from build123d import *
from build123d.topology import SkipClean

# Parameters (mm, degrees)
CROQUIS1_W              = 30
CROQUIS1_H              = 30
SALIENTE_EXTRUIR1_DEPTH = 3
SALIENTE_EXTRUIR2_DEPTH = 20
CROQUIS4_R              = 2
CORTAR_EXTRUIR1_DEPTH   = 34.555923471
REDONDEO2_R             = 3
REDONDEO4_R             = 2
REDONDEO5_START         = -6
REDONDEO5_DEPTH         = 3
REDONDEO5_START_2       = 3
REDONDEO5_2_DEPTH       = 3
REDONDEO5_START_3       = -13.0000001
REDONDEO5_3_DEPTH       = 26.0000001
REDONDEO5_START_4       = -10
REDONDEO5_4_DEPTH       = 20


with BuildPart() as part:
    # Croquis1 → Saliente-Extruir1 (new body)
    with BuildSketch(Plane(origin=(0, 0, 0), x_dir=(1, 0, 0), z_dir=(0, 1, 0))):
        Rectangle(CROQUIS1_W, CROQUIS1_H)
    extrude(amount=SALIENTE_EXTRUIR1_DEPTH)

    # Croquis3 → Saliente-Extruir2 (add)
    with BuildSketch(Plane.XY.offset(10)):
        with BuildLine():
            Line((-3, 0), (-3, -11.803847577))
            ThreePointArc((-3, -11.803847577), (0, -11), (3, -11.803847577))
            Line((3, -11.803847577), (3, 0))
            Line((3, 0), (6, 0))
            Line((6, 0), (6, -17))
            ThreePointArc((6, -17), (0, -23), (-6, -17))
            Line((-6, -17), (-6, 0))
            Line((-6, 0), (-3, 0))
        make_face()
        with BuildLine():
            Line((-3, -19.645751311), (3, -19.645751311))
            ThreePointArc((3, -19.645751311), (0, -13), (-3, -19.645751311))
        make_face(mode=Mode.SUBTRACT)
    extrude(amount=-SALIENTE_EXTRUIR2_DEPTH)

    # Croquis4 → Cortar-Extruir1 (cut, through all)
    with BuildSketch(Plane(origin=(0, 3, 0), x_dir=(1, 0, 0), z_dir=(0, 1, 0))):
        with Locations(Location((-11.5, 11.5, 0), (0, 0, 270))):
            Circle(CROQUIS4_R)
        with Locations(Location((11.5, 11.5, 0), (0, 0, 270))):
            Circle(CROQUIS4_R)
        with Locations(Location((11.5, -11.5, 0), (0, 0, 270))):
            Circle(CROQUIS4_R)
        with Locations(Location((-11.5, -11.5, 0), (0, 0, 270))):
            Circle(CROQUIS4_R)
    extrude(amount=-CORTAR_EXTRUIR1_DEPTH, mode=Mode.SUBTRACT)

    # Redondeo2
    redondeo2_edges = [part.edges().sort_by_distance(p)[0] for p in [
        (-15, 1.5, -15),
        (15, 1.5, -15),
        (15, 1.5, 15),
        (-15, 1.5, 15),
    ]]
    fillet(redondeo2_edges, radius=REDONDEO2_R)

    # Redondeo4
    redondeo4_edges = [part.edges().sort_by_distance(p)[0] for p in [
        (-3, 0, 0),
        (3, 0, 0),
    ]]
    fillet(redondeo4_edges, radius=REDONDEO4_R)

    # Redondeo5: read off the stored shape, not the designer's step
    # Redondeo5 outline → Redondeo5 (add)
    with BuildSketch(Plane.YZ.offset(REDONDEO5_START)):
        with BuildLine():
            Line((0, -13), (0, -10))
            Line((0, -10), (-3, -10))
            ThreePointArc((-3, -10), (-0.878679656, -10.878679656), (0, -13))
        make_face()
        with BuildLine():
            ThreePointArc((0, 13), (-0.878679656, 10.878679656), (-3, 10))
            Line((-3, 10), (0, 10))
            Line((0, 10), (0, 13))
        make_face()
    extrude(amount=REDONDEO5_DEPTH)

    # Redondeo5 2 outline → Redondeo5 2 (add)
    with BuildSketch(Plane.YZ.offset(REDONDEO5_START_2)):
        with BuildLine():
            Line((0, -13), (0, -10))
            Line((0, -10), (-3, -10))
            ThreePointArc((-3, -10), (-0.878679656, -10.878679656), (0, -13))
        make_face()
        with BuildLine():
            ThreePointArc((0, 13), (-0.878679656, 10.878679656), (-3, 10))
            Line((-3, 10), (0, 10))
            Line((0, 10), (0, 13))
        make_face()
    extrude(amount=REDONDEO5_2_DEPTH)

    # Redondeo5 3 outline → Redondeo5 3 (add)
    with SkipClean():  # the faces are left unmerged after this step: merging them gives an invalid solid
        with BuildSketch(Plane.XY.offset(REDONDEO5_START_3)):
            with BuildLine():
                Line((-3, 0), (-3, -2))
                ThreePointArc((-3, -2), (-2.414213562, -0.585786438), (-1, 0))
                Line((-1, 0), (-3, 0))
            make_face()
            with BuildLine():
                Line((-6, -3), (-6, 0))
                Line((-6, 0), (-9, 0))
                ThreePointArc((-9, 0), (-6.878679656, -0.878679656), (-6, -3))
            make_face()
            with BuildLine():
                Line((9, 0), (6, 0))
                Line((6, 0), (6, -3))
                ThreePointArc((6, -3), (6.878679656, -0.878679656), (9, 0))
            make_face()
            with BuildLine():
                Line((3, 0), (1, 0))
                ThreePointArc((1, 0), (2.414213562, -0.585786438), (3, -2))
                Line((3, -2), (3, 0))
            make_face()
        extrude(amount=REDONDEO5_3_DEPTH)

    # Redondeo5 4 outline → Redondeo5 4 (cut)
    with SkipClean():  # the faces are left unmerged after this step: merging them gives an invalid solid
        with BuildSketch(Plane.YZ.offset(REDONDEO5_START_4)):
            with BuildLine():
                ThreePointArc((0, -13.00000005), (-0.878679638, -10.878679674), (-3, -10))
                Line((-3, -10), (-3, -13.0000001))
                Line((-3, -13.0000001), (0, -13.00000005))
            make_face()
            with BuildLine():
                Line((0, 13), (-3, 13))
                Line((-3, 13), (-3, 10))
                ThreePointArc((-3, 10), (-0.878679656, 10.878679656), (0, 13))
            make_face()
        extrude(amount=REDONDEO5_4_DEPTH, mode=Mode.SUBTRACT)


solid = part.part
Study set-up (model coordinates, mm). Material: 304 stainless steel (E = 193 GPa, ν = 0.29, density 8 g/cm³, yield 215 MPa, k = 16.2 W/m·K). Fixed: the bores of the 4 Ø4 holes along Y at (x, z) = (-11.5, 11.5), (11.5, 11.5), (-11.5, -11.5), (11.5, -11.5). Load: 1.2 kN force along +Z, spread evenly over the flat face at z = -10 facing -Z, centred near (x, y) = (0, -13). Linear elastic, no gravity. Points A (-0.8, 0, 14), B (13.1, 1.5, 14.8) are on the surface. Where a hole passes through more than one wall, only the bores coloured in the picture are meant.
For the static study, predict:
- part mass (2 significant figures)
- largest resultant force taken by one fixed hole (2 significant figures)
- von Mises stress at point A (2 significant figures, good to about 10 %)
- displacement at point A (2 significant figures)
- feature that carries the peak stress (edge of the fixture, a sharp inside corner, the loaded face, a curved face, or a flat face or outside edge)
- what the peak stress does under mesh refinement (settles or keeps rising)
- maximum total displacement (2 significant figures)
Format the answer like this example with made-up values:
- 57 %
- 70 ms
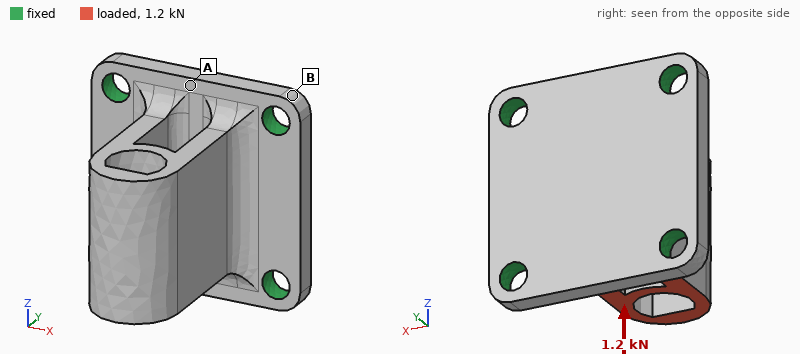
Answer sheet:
- 45 g
- 530 N
- 27 MPa
- 4.1 µm
- edge of the fixture
- keeps rising
- 13 µm
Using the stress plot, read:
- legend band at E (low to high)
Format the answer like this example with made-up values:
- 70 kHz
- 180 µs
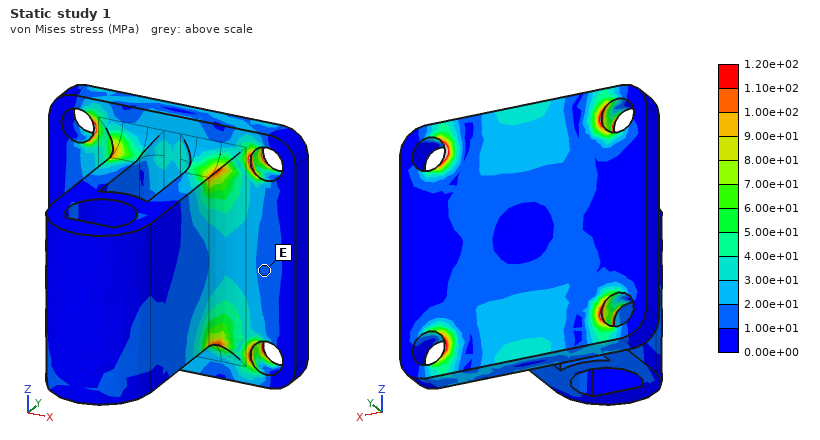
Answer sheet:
- 1.00e+01 to 2.00e+01 MPa
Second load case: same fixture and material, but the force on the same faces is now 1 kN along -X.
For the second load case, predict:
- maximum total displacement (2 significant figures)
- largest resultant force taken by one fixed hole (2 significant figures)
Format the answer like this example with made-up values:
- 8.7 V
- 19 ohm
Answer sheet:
- 33 µm
- 560 N
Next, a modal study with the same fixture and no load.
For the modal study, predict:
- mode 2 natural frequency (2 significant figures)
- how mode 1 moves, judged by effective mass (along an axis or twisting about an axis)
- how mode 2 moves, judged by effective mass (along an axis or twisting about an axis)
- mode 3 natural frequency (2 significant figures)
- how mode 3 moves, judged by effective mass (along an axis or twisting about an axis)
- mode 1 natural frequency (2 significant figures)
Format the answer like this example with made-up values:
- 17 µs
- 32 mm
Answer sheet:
- 12 kHz
- along X
- along Z
- 17 kHz
- along Y
- 8300 Hz
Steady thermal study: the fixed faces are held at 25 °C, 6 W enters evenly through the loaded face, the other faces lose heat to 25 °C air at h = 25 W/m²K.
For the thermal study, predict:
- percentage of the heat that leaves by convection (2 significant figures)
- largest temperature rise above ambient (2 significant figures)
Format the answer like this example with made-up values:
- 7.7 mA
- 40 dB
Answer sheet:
- 34 %
- 58 K
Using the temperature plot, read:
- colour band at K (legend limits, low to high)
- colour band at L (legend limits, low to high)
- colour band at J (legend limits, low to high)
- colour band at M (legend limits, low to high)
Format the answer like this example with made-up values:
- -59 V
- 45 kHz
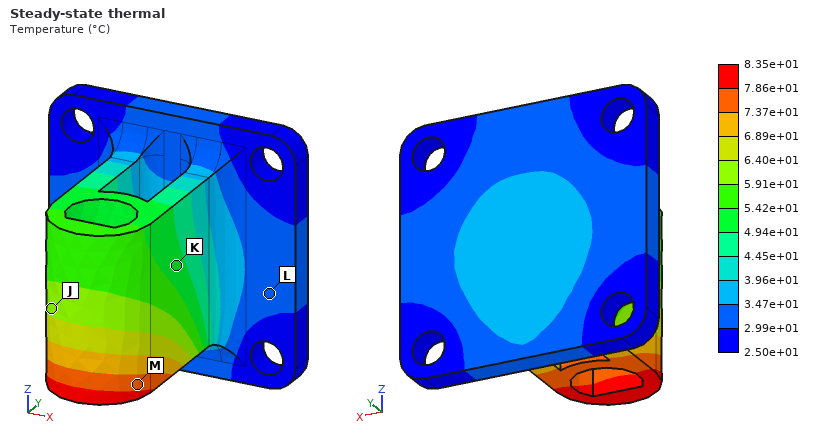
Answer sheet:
- 4.94e+01 to 5.42e+01 °C
- 2.99e+01 to 3.47e+01 °C
- 5.91e+01 to 6.40e+01 °C
- 7.37e+01 to 7.86e+01 °C
